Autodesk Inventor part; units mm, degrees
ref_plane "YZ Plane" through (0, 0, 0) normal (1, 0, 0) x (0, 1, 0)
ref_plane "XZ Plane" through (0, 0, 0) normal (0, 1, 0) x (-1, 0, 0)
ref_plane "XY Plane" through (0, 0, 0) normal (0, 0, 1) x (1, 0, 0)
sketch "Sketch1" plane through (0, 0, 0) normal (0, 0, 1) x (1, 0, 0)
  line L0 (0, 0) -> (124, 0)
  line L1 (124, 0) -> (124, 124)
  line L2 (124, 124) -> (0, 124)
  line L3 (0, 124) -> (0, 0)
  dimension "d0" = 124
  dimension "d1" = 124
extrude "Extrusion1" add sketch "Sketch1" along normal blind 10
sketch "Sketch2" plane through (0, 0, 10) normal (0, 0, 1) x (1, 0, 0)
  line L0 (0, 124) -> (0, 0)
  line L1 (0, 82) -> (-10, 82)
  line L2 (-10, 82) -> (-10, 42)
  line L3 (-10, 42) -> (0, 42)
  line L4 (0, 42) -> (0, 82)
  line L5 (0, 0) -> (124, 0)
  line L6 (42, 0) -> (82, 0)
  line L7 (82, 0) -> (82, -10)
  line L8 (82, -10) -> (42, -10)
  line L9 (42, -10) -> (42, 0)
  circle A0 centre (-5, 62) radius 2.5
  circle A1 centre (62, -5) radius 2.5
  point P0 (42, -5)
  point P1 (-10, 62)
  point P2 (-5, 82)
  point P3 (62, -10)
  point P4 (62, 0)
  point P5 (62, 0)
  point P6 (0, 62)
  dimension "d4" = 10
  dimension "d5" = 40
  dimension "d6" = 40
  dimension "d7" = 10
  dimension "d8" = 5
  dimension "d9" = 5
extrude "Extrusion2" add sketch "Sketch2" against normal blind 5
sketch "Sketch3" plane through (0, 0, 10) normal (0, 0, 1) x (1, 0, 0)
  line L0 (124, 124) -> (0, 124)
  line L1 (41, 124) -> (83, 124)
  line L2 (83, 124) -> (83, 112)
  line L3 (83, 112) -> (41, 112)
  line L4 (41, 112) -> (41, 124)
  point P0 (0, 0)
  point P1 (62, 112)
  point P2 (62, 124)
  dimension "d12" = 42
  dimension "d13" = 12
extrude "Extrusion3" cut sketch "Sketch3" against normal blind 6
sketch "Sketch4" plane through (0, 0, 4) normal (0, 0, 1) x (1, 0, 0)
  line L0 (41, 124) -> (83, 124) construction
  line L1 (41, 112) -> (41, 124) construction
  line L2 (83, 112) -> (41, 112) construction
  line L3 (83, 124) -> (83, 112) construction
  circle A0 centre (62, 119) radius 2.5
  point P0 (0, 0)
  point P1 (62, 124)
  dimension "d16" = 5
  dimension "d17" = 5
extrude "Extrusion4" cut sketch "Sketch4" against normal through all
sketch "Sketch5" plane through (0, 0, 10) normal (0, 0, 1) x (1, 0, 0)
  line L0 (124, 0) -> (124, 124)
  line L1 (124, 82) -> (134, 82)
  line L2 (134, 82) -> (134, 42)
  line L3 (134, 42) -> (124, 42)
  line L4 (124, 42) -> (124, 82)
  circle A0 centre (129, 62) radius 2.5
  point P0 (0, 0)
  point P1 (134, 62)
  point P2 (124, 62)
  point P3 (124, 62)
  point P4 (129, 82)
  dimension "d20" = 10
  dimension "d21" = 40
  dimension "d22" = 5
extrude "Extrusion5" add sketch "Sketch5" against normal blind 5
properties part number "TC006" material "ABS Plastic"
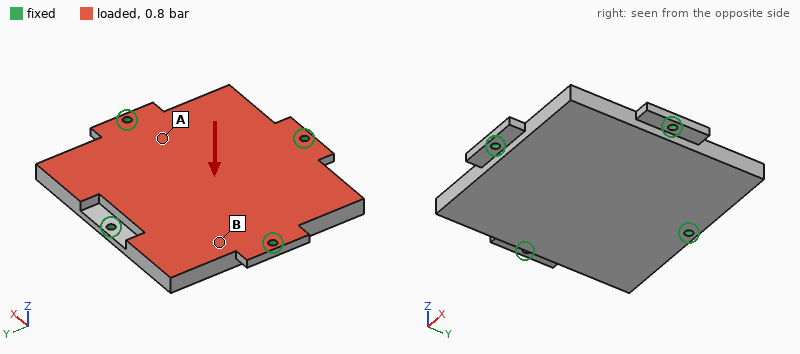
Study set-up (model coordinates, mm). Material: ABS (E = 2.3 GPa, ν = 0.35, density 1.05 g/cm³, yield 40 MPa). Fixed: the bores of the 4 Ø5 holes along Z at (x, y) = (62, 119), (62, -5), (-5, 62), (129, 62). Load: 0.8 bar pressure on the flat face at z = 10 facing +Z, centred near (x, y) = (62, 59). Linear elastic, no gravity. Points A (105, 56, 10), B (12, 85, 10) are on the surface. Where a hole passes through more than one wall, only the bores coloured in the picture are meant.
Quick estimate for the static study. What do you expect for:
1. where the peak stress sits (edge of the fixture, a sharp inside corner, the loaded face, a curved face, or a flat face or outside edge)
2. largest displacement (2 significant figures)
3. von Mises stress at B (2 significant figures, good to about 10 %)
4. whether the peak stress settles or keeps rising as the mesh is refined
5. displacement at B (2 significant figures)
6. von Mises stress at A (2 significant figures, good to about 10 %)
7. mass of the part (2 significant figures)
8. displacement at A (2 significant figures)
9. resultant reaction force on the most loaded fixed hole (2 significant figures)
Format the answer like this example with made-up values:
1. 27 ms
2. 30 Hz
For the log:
1. edge of the fixture
2. 0.36 mm
3. 3.5 MPa
4. keeps rising
5. 0.21 mm
6. 1.5 MPa
7. 160 g
8. 0.22 mm
9. 440 N
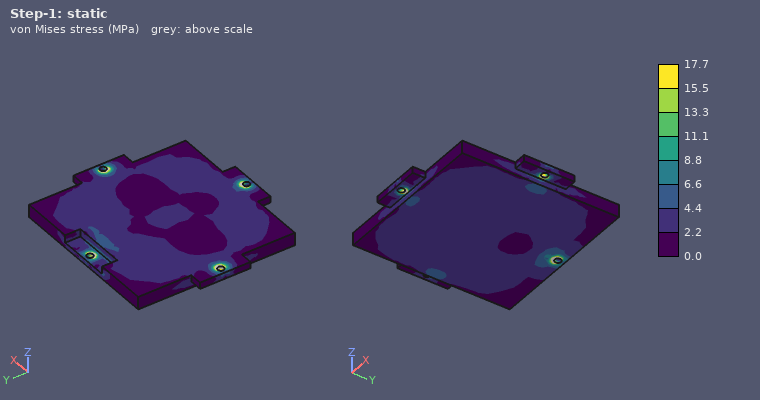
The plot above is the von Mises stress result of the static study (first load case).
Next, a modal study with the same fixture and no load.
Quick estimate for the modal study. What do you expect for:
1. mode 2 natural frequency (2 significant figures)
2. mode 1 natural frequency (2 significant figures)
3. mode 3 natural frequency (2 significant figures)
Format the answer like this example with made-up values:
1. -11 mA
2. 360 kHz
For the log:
1. 840 Hz
2. 730 Hz
3. 850 Hz
